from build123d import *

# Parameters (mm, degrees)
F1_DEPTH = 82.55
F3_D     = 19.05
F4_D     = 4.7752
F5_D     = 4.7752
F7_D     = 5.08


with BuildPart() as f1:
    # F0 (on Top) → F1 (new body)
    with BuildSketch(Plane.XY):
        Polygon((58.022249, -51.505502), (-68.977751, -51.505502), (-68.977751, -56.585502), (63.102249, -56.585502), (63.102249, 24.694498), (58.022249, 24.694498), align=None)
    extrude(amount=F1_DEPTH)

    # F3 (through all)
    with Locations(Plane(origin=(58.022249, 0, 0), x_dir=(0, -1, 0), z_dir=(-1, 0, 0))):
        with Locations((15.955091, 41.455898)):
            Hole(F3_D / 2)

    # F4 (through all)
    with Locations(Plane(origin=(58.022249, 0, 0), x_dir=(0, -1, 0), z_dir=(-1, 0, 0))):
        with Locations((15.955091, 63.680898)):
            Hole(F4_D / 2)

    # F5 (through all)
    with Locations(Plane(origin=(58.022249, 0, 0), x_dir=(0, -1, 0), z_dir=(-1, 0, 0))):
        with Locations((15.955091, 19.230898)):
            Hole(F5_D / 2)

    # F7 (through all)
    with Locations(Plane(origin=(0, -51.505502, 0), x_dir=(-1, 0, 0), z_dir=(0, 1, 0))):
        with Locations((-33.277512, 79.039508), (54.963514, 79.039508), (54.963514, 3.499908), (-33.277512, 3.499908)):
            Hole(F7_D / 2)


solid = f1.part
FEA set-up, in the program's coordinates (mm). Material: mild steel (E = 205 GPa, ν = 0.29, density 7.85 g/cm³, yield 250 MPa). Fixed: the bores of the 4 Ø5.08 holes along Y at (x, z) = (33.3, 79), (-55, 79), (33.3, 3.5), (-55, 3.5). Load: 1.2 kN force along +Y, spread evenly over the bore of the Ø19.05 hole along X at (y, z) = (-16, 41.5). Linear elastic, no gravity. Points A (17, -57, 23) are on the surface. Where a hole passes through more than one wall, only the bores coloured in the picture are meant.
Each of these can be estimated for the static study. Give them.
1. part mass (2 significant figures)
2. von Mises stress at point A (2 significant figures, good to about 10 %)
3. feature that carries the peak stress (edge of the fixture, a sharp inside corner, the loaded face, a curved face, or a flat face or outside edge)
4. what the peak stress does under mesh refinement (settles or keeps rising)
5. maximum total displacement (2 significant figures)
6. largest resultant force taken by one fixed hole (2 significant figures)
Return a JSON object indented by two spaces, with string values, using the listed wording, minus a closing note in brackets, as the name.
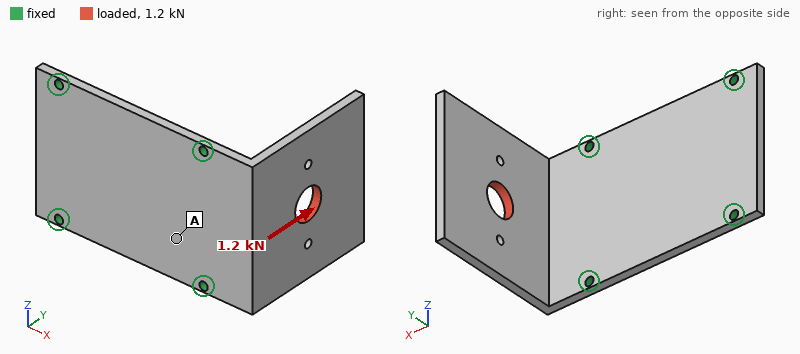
{
  "part mass": "670 g",
  "von Mises stress at point A": "17 MPa",
  "feature that carries the peak stress": "edge of the fixture",
  "what the peak stress does under mesh refinement": "keeps rising",
  "maximum total displacement": "0.26 mm",
  "largest resultant force taken by one fixed hole": "660 N"
}
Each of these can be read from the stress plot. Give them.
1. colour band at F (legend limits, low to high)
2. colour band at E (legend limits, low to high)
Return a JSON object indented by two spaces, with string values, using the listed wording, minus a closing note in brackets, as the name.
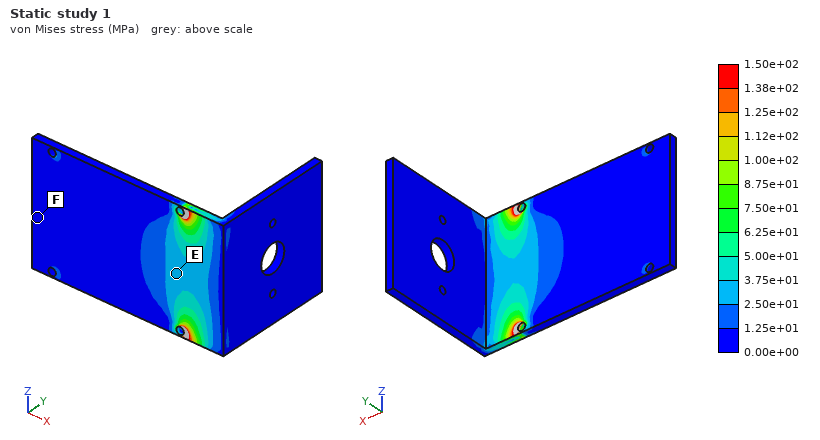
{
  "colour band at F": "0.00e+00 to 1.25e+01 MPa",
  "colour band at E": "2.50e+01 to 3.75e+01 MPa"
}
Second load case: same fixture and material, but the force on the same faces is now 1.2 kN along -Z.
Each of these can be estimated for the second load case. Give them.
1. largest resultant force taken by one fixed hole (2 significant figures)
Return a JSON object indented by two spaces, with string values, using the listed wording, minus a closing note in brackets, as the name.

{
  "largest resultant force taken by one fixed hole": "980 N"
}
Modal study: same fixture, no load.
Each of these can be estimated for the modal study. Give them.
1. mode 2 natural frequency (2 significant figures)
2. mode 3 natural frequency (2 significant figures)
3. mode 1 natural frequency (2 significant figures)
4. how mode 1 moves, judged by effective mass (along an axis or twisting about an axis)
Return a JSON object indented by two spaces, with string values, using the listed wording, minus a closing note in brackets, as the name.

{
  "mode 2 natural frequency": "1100 Hz",
  "mode 3 natural frequency": "1600 Hz",
  "mode 1 natural frequency": "420 Hz",
  "how mode 1 moves, judged by effective mass": "along X"
}
